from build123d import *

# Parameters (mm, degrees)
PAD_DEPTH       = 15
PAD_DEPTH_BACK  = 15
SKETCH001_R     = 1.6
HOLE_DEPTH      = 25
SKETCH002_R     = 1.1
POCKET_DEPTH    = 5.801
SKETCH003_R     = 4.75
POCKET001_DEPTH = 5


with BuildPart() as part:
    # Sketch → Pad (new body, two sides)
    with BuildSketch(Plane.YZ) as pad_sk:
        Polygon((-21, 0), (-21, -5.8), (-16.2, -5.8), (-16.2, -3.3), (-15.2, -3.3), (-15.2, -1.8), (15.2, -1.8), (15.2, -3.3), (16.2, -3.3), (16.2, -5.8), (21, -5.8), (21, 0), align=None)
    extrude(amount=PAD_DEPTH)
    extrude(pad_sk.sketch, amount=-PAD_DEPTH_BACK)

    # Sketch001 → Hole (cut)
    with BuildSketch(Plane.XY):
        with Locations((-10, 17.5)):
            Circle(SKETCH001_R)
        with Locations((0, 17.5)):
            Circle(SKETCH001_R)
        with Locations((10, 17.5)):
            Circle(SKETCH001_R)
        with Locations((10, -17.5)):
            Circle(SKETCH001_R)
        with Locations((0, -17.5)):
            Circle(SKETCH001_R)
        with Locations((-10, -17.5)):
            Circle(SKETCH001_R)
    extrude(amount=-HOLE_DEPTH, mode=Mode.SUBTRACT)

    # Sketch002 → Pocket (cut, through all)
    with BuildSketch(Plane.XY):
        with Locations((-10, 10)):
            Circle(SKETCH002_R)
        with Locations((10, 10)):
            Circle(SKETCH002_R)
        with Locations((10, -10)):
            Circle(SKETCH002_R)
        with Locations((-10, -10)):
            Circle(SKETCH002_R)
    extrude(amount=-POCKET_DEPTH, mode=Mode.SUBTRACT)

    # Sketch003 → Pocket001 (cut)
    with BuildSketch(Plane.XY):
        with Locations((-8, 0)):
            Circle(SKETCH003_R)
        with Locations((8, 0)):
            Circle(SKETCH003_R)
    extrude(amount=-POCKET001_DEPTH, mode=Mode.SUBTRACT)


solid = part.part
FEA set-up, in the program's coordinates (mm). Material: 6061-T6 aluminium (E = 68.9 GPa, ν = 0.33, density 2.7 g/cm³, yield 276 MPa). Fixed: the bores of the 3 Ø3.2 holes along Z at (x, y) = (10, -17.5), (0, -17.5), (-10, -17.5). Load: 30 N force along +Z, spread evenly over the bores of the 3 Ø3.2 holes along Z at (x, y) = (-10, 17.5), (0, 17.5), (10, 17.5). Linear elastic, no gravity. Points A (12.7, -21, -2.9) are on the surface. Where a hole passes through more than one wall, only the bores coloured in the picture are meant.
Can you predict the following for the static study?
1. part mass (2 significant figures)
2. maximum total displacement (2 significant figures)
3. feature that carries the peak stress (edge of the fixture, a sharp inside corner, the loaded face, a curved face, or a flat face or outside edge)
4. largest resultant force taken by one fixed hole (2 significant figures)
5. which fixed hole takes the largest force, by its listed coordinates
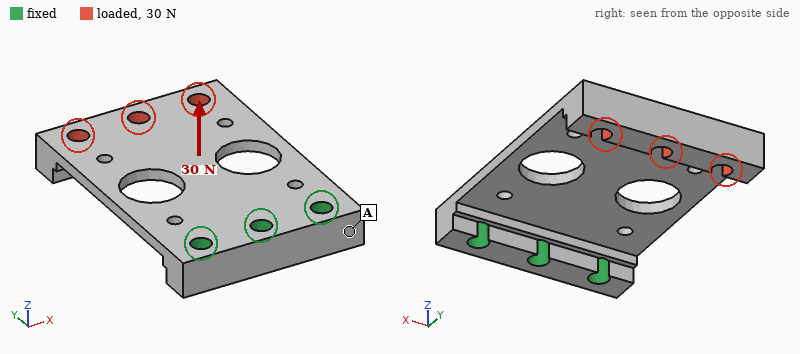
8.0 g
0.60 mm
a curved face
18 N
(0, -17.5)
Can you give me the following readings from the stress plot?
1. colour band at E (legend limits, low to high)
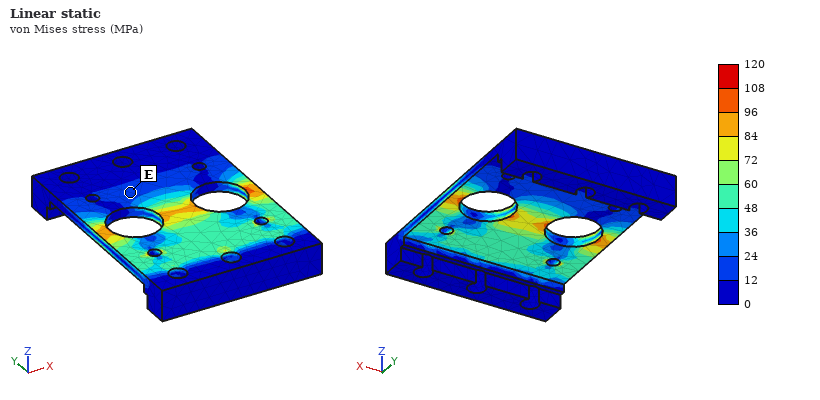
12 to 24 MPa
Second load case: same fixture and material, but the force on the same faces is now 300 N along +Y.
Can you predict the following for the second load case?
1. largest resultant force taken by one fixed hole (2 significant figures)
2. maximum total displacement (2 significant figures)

100 N
0.54 mm
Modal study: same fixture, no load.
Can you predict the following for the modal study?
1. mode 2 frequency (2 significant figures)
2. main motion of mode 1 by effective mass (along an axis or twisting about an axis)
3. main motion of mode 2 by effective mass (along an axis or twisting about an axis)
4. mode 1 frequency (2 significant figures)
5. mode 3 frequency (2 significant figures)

2300 Hz
along Z
twisting about Y
700 Hz
5500 Hz
